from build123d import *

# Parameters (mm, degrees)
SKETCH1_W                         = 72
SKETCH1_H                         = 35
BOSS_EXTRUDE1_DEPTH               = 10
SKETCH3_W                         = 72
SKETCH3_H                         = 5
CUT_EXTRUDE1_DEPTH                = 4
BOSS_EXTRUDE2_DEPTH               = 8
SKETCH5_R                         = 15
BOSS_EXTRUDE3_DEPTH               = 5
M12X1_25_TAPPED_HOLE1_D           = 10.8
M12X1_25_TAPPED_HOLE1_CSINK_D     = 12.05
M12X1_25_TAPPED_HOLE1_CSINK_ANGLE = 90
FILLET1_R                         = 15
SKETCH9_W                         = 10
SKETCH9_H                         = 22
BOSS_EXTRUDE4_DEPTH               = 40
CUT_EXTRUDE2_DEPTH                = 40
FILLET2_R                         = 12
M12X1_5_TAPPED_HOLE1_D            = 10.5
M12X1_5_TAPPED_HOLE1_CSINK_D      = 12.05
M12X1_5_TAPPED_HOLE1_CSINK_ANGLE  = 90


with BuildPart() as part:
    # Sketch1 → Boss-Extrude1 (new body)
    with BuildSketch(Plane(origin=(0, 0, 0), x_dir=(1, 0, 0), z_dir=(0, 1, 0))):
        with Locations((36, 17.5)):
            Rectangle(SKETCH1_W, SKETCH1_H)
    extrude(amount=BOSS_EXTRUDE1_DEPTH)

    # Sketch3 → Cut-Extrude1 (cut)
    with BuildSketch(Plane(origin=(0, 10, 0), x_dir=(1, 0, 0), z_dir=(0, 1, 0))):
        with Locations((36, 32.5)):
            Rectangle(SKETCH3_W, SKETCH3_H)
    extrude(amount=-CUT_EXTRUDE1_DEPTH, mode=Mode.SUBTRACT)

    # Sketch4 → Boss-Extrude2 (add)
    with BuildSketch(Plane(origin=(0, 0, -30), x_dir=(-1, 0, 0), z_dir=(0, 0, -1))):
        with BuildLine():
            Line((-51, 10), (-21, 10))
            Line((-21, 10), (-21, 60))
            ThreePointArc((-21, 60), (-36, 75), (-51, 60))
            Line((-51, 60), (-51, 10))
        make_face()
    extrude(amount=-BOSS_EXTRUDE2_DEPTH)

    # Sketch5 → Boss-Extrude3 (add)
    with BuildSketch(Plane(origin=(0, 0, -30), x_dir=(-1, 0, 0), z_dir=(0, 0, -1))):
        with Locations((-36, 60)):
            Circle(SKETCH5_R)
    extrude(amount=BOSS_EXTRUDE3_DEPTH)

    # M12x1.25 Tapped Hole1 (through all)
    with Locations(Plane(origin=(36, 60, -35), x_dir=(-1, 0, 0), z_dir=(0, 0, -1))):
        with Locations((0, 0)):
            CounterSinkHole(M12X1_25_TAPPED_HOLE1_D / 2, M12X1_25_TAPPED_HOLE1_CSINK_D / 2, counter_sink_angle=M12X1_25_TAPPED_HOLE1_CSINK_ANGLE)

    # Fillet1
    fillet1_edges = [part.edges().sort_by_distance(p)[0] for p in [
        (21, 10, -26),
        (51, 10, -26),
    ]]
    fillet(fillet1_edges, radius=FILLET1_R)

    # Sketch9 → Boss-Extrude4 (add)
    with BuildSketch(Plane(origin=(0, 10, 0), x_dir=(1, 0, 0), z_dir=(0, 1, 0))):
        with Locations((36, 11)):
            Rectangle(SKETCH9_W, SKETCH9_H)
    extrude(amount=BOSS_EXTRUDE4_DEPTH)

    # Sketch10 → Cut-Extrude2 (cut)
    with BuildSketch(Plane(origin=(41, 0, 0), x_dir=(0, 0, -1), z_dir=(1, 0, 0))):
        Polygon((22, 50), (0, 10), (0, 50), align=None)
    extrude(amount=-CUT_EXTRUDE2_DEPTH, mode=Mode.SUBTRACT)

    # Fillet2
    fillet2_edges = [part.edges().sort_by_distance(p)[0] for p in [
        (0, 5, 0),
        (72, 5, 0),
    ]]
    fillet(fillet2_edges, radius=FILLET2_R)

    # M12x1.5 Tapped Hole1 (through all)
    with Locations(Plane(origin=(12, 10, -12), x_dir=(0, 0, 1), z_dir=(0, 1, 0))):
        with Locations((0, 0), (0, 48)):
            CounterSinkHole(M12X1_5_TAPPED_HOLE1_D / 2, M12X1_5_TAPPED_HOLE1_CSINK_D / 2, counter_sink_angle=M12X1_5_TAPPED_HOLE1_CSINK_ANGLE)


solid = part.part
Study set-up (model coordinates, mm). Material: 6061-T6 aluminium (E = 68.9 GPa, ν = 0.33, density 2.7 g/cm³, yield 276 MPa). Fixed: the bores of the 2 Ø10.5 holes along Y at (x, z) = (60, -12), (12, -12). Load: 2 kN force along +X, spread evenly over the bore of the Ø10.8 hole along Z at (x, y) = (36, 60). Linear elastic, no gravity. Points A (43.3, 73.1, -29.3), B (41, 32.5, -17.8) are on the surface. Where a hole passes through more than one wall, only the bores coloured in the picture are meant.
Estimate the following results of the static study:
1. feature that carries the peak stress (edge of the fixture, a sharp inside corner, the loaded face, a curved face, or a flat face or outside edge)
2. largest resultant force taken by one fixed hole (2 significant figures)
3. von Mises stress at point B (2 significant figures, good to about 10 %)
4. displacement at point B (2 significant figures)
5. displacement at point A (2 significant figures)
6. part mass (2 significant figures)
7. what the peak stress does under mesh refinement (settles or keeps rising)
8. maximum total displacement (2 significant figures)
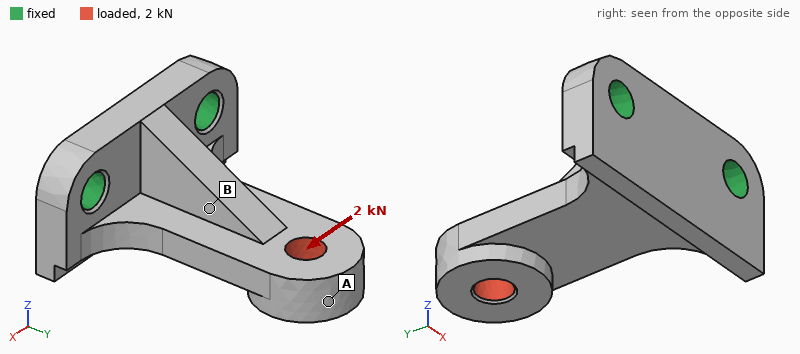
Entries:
edge of the fixture
2.8 kN
16 MPa
0.030 mm
0.13 mm
120 g
keeps rising
0.14 mm
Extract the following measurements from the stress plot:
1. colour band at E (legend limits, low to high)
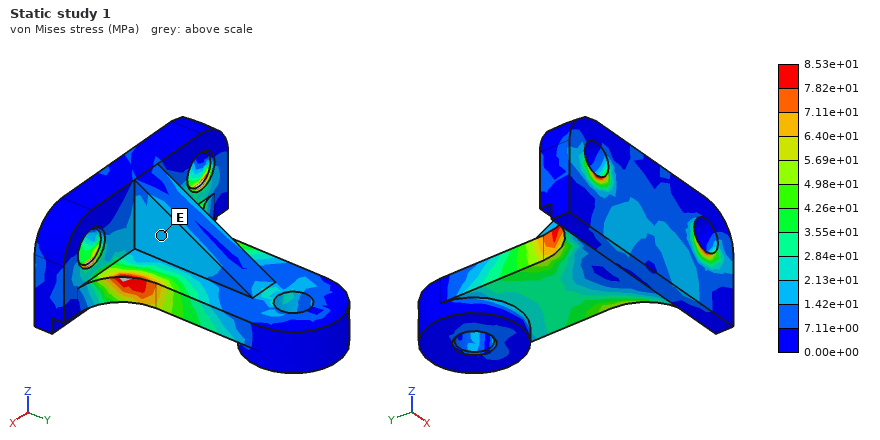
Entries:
1.42e+01 to 2.13e+01 MPa
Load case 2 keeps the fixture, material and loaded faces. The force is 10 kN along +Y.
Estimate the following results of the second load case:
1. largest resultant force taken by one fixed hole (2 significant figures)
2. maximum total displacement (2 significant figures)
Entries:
5.2 kN
0.38 mm
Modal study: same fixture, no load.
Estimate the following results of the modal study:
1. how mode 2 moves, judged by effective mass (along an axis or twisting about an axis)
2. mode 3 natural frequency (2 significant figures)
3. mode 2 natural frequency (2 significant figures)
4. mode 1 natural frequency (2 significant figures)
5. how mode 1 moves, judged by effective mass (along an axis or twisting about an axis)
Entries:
along X
7600 Hz
4300 Hz
2500 Hz
along Z
